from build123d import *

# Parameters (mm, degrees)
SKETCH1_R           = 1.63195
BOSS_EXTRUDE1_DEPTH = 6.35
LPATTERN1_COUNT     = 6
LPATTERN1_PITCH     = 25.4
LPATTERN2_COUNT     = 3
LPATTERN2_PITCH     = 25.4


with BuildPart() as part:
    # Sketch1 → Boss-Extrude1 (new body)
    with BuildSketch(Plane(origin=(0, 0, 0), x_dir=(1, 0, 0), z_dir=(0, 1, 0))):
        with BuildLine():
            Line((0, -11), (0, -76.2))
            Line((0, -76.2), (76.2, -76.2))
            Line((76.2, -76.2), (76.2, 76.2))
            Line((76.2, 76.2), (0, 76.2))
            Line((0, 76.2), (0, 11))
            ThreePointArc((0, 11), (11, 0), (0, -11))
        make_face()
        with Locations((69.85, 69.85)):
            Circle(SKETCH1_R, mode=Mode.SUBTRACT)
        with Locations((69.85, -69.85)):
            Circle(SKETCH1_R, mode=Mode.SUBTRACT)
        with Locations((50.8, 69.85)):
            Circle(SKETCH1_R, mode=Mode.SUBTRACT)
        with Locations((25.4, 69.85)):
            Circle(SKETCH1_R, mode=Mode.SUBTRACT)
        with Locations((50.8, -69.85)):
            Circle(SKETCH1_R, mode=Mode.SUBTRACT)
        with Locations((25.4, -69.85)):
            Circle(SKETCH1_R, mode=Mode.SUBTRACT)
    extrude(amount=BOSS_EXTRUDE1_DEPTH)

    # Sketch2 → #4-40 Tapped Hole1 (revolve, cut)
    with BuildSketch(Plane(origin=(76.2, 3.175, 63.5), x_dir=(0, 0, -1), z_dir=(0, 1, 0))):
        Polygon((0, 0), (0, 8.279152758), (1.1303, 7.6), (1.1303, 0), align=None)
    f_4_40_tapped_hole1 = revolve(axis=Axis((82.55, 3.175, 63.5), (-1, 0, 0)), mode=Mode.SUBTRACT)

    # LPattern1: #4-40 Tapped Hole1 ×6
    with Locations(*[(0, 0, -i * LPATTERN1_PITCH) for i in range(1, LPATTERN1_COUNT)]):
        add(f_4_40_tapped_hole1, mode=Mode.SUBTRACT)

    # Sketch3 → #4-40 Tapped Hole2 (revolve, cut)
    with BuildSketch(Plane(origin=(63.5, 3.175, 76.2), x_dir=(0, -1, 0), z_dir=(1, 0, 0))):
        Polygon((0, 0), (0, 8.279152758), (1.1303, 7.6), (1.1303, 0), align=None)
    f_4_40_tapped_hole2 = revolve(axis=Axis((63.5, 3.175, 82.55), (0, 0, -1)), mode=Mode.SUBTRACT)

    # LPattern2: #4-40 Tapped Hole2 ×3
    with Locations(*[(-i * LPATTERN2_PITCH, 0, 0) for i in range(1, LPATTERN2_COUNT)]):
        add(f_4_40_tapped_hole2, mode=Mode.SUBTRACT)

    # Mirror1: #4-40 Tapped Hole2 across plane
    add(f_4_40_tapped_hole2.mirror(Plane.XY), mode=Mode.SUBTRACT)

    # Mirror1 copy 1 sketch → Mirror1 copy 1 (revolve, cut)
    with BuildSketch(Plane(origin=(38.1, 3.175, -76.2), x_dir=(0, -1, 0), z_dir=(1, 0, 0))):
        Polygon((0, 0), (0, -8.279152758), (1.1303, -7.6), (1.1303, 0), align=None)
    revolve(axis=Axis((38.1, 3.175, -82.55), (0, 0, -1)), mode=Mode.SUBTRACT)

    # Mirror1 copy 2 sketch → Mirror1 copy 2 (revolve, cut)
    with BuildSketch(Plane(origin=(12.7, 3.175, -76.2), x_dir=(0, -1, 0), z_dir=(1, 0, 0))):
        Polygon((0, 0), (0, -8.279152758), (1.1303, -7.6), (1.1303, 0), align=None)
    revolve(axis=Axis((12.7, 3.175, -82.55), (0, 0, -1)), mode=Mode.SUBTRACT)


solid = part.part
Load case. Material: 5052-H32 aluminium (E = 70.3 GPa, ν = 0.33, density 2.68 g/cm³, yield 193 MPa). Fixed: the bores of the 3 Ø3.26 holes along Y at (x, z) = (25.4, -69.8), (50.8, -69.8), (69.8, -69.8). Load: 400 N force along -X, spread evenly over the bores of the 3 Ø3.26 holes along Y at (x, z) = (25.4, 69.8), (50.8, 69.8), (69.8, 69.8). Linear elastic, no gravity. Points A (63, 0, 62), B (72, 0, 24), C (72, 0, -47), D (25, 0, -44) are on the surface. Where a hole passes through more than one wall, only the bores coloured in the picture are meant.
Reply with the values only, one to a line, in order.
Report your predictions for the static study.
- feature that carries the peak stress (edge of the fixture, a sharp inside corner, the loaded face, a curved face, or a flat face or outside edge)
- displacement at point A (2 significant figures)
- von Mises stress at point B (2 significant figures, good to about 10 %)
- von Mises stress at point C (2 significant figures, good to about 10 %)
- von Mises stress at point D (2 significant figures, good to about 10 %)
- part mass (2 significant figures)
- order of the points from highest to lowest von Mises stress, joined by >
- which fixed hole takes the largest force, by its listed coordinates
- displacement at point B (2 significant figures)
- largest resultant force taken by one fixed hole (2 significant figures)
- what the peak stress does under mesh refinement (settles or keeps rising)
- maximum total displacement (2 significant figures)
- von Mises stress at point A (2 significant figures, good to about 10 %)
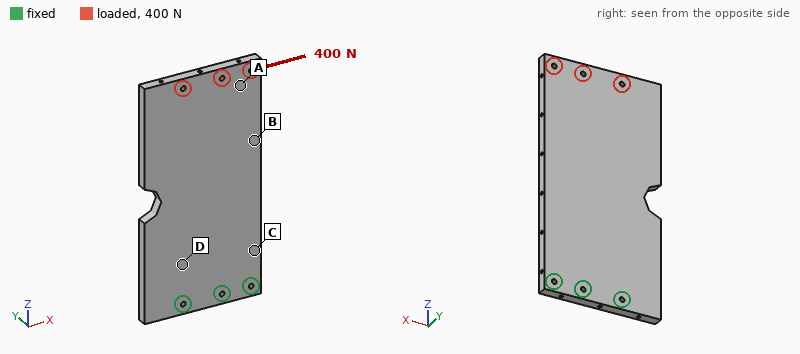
edge of the fixture
43 µm
3.1 MPa
8.8 MPa
5.7 MPa
190 g
C > D > B > A
(25.4, -69.8)
29 µm
1.3 kN
keeps rising
51 µm
1.8 MPa
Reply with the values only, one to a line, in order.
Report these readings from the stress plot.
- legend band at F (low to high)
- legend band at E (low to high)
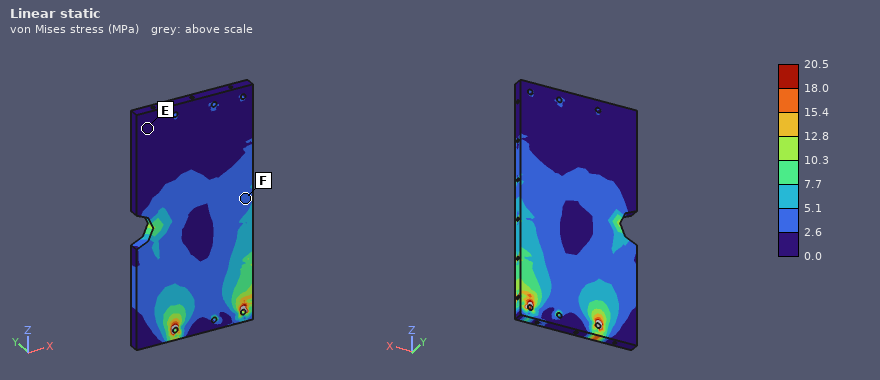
2.6 to 5.1 MPa
0.0 to 2.6 MPa
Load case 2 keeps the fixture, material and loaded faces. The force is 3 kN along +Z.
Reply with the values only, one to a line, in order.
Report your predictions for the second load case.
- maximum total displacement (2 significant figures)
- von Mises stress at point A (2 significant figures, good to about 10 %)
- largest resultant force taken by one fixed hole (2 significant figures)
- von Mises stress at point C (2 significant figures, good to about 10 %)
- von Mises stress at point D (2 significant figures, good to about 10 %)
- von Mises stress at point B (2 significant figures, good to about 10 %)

28 µm
7.8 MPa
1.0 kN
9.8 MPa
5.2 MPa
10 MPa
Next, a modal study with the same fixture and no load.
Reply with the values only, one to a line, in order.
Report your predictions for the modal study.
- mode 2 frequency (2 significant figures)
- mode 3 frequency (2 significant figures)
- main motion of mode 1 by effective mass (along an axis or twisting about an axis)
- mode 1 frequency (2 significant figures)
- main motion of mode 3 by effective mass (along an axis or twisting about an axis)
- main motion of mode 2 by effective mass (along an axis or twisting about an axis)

960 Hz
1500 Hz
along Y
240 Hz
along Y
twisting about Z
